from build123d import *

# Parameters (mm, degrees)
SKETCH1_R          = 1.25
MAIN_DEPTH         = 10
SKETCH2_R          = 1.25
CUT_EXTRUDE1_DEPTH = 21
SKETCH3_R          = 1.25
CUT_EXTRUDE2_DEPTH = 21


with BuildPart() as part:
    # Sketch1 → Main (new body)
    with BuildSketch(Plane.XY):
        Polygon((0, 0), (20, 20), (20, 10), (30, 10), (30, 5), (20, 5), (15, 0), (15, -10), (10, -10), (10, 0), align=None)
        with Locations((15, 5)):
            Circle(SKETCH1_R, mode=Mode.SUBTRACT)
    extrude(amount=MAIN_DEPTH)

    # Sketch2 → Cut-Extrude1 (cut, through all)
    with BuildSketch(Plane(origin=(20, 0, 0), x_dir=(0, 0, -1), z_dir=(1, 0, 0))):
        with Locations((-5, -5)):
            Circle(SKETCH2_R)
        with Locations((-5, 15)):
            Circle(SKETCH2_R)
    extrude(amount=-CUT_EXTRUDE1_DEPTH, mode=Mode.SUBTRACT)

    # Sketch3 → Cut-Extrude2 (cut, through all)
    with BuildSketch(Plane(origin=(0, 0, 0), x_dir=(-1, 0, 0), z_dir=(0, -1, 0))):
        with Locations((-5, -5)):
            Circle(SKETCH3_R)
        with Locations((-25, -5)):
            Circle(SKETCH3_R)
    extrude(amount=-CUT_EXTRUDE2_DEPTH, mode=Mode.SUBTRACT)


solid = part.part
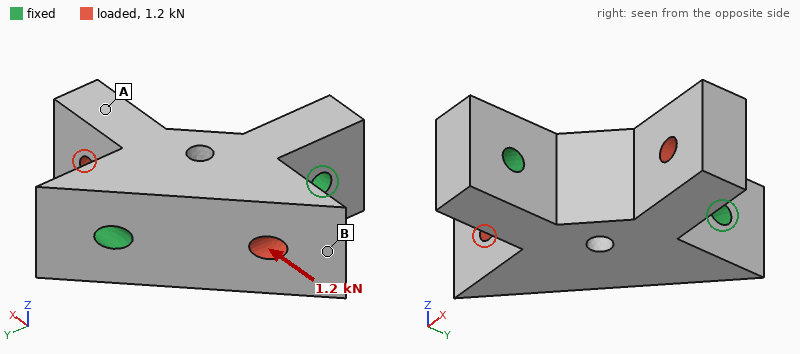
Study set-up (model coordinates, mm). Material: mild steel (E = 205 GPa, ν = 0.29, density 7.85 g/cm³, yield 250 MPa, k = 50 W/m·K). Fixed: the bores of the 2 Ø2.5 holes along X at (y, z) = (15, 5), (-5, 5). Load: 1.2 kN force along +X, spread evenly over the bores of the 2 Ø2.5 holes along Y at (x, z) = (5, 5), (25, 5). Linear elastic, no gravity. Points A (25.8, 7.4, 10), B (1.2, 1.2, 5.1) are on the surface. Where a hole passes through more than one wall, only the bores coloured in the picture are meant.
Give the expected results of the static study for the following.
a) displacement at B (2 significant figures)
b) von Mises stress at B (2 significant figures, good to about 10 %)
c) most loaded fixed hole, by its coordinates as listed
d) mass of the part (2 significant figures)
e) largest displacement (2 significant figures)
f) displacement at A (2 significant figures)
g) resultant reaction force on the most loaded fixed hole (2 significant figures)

2.2 µm
19 MPa
(15, 5)
21 g
2.7 µm
1.8 µm
670 N
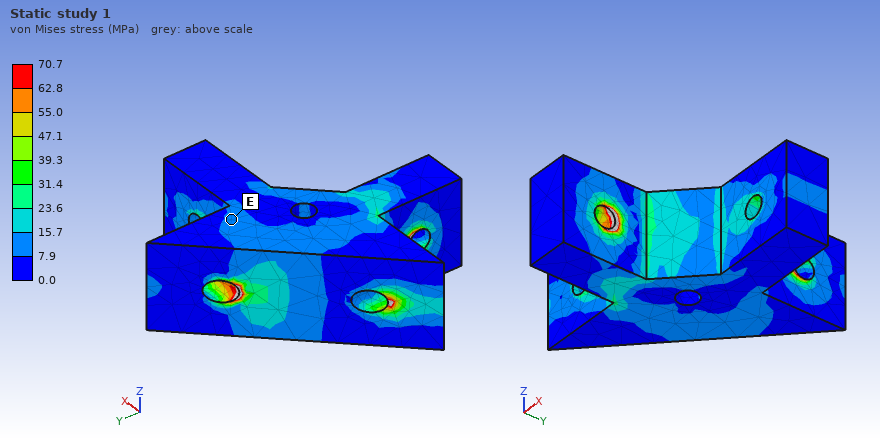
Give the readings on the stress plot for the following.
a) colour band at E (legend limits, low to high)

7.9 to 15.7 MPa
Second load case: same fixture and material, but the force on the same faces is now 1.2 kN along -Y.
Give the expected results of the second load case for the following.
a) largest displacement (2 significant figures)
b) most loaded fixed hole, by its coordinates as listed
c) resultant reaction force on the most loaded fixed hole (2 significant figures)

8.5 µm
(15, 5)
740 N
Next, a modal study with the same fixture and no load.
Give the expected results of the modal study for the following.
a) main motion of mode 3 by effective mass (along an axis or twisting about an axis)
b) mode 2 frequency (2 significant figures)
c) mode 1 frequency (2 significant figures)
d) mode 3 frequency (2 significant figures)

along Z
24 kHz
18 kHz
28 kHz
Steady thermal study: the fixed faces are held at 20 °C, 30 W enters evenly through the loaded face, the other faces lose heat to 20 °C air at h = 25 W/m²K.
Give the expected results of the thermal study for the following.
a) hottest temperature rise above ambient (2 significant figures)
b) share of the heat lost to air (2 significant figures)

81 K
4.6 %
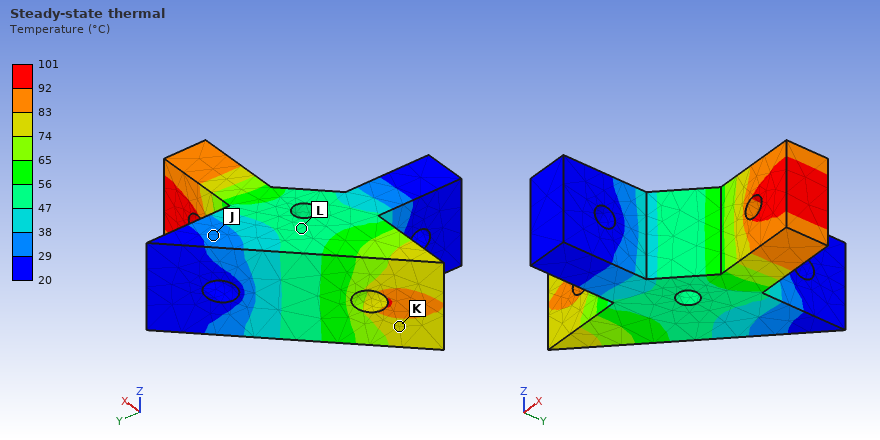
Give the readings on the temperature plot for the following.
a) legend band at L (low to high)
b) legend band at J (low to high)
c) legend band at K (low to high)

47 to 56 °C
29 to 38 °C
74 to 83 °C
